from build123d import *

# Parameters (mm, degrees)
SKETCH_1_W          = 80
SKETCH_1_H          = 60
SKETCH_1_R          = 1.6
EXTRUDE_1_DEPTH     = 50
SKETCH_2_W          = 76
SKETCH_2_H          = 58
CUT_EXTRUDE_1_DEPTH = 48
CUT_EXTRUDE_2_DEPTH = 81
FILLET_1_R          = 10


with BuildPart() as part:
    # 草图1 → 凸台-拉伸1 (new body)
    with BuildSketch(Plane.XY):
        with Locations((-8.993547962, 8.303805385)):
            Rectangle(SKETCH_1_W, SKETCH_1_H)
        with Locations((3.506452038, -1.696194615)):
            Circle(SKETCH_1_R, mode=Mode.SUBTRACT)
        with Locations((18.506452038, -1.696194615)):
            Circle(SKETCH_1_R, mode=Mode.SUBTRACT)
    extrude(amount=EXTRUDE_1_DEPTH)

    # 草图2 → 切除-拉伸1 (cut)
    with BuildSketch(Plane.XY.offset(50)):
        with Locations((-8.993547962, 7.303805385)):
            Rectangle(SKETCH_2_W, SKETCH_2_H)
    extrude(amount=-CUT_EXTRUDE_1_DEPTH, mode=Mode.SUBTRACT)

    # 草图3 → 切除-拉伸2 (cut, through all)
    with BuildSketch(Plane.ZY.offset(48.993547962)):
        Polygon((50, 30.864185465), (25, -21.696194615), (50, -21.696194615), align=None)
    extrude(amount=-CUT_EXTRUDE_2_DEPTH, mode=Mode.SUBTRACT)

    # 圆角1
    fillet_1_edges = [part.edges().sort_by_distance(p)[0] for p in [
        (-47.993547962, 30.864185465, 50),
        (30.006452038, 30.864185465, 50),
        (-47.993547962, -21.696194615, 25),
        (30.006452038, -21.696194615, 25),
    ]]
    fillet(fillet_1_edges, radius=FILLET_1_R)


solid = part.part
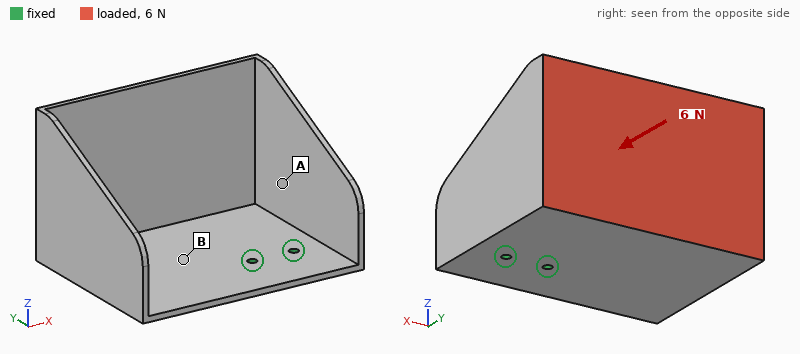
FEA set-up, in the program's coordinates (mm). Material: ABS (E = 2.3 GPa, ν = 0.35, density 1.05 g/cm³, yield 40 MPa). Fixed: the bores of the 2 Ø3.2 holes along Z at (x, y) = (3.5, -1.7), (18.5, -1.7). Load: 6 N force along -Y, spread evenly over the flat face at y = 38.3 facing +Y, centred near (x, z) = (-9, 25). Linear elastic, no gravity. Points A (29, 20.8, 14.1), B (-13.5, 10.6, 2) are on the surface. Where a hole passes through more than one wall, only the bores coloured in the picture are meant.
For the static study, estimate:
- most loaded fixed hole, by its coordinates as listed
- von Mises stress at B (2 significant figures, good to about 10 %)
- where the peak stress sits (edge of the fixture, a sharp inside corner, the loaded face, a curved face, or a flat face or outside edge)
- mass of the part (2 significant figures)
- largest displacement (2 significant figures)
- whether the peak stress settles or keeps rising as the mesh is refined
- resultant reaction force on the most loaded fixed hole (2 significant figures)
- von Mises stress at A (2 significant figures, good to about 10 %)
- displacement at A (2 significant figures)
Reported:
(3.5, -1.7)
0.88 MPa
edge of the fixture
27 g
1.1 mm
keeps rising
10 N
0.37 MPa
0.27 mm
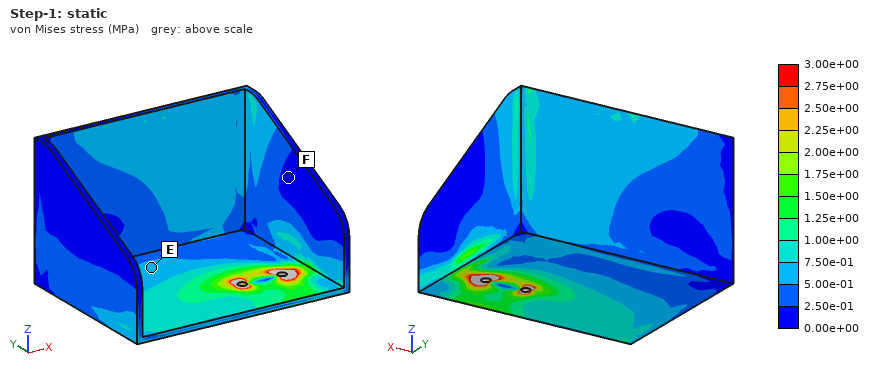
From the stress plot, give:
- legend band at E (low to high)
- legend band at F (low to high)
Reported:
5.00e-01 to 7.50e-01 MPa
0.00e+00 to 2.50e-01 MPa
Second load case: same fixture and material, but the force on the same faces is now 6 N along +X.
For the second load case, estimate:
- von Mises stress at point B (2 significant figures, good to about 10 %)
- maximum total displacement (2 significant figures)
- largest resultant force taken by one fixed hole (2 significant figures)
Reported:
0.61 MPa
1.2 mm
15 N
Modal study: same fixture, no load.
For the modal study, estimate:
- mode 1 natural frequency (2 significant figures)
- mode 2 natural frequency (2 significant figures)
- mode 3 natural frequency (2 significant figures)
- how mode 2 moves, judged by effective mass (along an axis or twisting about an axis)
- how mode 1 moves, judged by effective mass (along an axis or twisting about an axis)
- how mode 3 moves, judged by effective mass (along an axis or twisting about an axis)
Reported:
77 Hz
110 Hz
190 Hz
along Y
along Z
along Z
